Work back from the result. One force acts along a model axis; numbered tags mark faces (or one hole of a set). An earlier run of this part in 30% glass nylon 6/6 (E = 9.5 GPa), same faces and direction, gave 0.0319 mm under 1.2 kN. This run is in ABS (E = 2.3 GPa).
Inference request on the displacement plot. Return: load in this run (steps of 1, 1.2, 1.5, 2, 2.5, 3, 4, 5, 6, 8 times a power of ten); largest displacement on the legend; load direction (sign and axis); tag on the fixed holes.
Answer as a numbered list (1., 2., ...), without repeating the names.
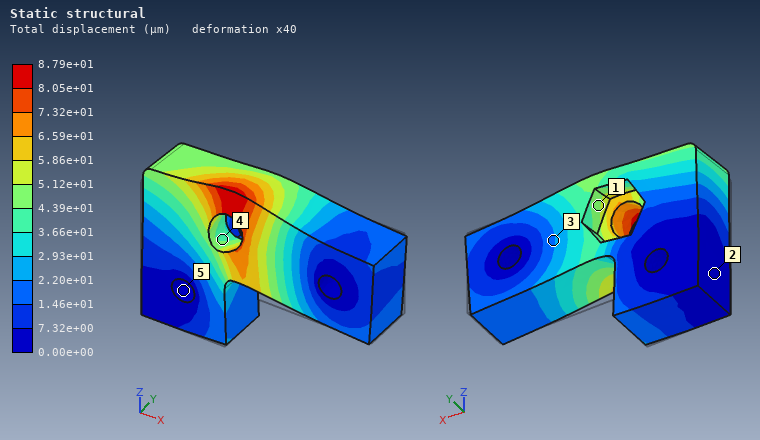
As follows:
1. 800 N
2. 8.79e+01 µm
3. +Z
4. 5
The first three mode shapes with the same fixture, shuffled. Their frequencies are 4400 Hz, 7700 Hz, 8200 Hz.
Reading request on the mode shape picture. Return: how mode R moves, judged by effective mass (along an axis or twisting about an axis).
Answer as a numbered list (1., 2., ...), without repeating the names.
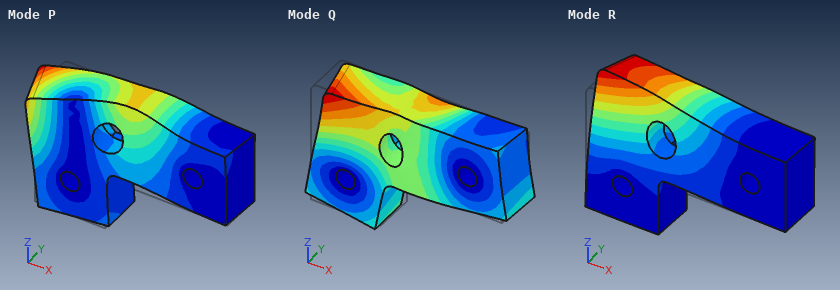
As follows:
1. along Y
